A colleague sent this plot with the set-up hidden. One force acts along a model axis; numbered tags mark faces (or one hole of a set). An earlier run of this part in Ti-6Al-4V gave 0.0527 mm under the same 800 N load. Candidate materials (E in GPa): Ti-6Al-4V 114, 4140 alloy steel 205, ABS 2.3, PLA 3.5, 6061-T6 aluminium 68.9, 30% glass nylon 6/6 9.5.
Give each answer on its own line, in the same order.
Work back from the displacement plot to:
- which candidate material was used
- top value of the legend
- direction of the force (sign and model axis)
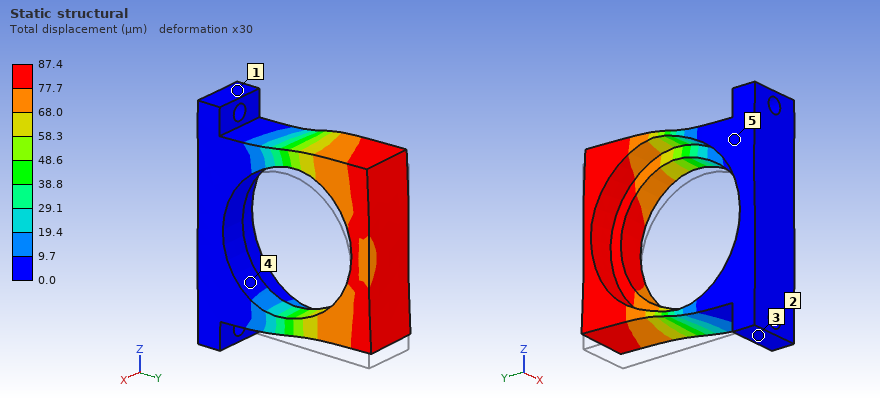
6061-T6 aluminium
87.4 µm
+Z
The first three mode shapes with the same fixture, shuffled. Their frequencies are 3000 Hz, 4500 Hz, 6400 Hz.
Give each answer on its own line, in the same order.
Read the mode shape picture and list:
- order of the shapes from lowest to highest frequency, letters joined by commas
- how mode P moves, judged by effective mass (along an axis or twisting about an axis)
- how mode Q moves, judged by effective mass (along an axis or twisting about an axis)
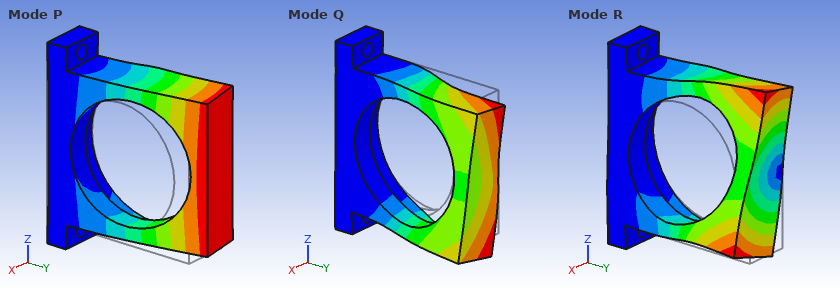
P, Q, R
along X
along Z
